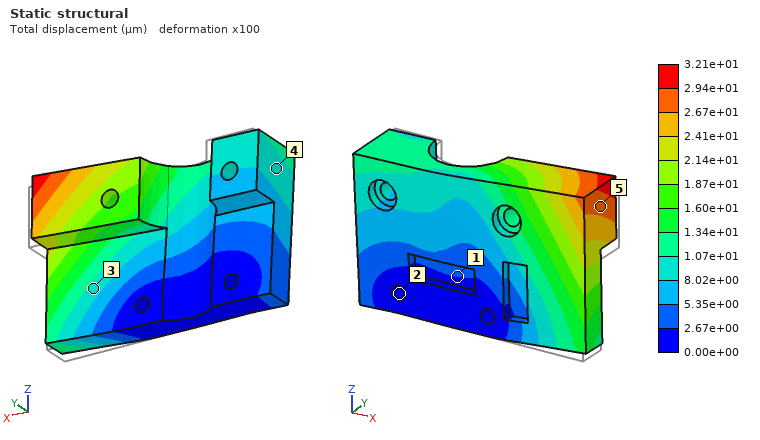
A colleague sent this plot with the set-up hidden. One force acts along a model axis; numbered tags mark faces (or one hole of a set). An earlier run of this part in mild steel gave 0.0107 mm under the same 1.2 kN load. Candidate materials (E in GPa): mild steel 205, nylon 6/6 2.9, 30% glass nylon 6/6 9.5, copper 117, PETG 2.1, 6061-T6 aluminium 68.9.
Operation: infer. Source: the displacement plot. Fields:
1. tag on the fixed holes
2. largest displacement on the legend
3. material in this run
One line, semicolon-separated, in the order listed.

2; 3.21e+01 µm; 6061-T6 aluminium
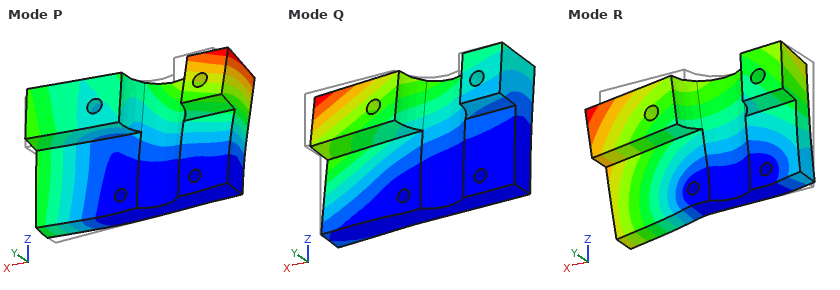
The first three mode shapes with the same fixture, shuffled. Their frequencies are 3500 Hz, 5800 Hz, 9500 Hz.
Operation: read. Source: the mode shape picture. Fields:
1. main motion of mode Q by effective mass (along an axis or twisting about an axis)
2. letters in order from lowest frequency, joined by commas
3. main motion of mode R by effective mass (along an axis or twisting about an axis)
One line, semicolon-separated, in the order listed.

along Y; Q, P, R; along X
